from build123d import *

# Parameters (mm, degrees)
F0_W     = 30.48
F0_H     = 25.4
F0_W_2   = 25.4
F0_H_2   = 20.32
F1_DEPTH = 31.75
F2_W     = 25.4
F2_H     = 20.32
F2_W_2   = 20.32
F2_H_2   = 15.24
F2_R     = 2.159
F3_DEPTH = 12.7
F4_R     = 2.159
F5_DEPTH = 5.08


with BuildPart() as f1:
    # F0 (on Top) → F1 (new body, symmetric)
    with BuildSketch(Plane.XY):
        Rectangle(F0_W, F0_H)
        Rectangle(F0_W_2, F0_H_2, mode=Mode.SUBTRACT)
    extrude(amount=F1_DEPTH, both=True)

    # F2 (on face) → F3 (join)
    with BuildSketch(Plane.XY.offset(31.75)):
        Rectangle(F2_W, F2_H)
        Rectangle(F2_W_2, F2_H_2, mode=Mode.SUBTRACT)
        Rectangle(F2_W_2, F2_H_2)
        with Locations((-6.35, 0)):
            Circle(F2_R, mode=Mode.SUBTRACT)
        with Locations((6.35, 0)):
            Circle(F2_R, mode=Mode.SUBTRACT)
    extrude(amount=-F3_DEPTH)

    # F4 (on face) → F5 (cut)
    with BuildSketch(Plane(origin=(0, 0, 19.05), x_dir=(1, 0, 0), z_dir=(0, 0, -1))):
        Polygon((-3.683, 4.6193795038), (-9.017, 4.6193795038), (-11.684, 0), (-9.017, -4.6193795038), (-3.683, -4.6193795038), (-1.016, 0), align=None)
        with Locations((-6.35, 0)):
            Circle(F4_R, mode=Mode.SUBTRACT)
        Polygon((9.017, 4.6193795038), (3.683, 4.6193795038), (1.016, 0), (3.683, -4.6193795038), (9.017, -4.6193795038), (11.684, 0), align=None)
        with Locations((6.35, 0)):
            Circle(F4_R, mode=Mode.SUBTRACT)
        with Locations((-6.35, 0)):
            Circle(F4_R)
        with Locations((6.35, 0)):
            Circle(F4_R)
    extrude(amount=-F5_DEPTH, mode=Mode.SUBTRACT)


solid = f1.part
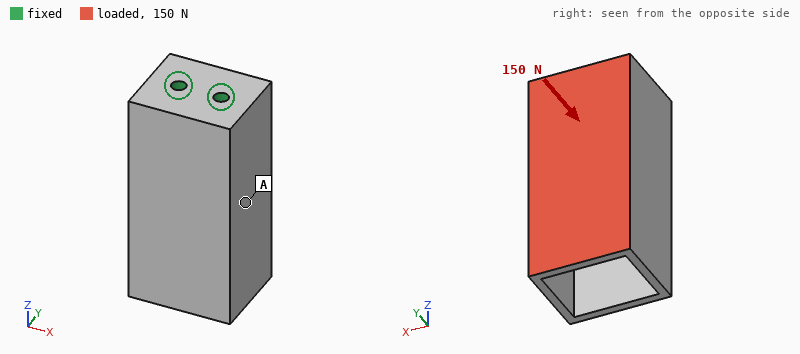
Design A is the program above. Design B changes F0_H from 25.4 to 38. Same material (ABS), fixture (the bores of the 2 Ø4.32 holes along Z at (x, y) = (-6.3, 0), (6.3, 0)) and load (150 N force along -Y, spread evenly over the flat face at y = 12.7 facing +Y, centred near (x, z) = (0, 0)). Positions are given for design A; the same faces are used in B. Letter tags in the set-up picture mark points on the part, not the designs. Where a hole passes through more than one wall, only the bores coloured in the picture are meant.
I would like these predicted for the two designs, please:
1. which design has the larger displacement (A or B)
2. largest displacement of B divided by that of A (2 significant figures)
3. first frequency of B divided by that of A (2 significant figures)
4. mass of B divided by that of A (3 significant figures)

A
0.71
0.67
2.11
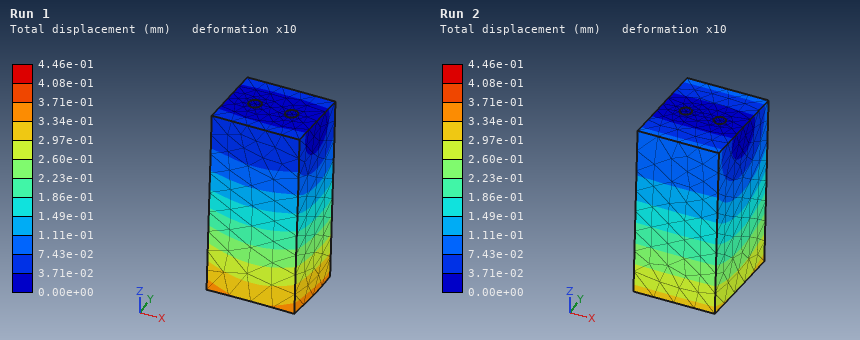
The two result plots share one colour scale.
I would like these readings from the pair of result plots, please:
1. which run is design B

Run 2
